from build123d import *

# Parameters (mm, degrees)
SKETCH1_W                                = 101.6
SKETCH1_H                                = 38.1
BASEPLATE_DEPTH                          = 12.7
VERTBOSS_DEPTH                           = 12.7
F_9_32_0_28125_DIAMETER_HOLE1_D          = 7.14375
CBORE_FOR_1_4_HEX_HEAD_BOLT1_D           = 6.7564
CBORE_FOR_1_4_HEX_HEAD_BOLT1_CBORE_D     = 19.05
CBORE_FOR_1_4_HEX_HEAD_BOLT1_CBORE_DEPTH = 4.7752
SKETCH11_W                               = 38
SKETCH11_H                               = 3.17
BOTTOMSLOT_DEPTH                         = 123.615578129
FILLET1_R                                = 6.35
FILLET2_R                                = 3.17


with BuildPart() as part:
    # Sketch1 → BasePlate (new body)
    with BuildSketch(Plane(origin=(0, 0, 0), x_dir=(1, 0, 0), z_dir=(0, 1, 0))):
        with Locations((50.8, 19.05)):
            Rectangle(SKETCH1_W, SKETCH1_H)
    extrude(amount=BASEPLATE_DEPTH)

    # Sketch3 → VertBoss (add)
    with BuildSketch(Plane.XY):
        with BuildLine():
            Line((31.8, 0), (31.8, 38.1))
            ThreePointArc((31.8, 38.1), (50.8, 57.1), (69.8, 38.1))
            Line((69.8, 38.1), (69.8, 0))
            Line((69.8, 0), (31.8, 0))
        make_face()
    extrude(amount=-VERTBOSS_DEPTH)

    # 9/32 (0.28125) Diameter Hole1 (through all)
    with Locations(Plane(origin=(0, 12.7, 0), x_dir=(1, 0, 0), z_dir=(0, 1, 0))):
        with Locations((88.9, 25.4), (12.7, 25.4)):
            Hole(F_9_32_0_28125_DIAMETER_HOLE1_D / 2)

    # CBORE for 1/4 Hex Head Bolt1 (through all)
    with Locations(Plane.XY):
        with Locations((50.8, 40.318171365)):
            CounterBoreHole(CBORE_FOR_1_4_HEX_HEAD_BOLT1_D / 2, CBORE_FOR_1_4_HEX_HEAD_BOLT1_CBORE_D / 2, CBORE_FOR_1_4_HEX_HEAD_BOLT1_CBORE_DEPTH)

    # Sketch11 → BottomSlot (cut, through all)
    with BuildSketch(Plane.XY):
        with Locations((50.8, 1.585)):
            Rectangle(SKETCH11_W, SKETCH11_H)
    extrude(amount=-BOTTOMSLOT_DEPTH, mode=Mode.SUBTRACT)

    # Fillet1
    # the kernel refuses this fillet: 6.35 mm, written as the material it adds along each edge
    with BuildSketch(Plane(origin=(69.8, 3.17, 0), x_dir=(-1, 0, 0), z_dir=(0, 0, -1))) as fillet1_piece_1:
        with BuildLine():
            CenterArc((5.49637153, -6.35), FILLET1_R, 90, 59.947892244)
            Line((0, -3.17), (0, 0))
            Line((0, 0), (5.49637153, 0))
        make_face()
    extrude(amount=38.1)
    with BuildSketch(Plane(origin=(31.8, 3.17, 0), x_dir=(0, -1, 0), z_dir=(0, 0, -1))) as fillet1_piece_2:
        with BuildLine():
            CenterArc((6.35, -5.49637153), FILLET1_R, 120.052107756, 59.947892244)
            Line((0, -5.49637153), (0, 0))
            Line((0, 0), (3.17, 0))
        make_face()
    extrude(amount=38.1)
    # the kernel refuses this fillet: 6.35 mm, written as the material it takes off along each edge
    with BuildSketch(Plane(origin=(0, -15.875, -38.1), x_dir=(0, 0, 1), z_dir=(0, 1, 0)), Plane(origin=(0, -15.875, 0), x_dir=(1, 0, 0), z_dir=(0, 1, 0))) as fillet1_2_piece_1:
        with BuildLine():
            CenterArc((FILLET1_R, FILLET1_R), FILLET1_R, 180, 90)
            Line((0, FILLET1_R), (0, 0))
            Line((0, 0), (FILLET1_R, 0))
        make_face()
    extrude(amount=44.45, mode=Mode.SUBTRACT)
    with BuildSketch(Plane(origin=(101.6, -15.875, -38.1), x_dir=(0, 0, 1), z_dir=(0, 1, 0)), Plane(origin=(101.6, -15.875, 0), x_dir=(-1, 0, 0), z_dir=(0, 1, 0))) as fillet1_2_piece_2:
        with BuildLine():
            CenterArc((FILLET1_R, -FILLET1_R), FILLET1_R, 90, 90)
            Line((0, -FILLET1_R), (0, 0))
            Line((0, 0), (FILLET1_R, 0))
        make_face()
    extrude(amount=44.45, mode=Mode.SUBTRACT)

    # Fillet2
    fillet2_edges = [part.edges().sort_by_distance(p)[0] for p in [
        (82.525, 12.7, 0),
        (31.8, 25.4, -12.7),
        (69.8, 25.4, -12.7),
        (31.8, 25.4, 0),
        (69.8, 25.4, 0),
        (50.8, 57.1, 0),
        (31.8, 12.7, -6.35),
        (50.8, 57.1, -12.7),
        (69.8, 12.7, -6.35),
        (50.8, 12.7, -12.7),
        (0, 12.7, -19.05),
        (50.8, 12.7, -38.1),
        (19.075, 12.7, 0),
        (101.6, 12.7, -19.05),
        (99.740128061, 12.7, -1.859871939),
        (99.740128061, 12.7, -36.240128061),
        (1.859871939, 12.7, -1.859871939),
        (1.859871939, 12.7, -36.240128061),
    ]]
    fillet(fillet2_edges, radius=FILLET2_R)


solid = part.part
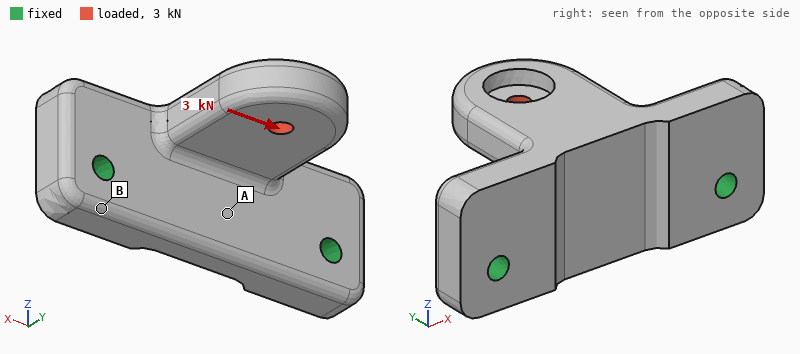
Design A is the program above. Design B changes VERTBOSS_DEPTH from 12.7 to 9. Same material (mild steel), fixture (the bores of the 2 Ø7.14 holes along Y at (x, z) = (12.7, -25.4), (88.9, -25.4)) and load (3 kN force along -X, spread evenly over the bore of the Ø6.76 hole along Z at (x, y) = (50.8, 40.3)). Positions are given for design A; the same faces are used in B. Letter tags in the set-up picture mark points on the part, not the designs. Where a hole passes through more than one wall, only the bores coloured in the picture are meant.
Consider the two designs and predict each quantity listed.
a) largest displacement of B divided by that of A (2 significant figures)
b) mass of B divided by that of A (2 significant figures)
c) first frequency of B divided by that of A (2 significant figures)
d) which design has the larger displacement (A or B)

1.4
0.91
0.98
B
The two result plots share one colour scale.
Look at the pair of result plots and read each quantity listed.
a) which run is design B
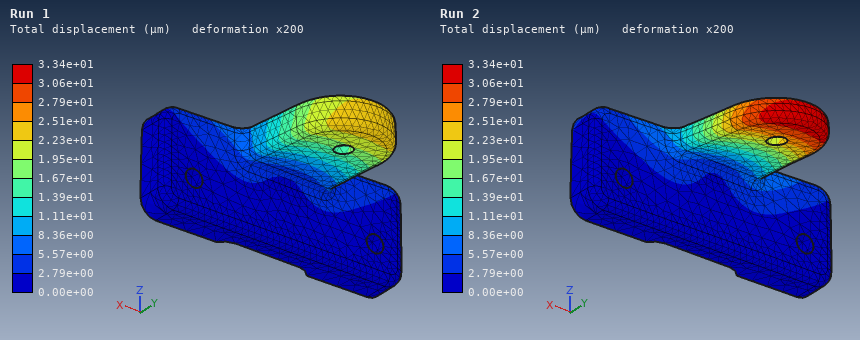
Run 2
